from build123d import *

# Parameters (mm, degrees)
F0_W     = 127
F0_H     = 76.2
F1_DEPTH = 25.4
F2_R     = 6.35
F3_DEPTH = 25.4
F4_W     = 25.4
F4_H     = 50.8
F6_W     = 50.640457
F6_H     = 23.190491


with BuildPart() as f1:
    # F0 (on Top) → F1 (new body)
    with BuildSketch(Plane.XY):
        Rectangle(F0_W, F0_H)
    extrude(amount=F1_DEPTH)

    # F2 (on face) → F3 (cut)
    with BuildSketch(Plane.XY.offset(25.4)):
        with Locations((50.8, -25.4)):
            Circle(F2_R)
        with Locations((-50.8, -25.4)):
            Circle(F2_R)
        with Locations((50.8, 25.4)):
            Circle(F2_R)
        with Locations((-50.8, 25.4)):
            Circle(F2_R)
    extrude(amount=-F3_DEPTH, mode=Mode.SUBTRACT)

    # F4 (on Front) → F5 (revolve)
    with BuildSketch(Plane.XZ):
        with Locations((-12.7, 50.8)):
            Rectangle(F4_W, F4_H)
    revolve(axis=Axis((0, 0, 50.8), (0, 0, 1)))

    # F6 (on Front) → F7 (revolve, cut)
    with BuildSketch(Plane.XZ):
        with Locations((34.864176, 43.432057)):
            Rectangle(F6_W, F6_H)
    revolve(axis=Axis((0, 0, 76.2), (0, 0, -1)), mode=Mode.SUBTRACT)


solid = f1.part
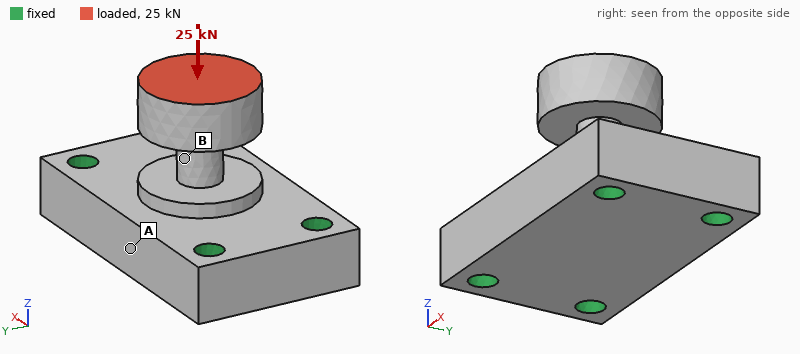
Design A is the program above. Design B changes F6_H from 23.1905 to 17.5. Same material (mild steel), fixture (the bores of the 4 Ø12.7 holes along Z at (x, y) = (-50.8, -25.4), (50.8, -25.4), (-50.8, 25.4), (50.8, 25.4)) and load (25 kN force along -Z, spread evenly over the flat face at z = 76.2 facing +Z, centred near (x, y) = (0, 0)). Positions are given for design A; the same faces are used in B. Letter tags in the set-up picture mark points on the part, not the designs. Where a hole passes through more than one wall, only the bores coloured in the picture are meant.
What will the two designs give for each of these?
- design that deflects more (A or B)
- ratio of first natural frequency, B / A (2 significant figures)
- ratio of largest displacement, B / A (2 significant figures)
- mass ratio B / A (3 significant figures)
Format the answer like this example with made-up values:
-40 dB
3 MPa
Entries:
A
1.1
0.88
1.03
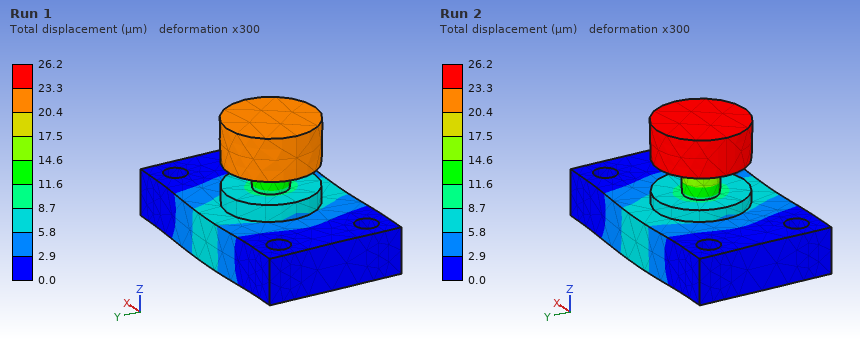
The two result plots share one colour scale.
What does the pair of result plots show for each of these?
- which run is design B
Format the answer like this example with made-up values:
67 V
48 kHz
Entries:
Run 1
